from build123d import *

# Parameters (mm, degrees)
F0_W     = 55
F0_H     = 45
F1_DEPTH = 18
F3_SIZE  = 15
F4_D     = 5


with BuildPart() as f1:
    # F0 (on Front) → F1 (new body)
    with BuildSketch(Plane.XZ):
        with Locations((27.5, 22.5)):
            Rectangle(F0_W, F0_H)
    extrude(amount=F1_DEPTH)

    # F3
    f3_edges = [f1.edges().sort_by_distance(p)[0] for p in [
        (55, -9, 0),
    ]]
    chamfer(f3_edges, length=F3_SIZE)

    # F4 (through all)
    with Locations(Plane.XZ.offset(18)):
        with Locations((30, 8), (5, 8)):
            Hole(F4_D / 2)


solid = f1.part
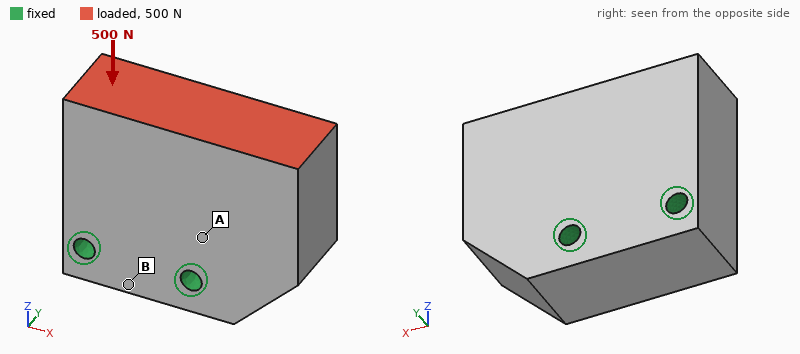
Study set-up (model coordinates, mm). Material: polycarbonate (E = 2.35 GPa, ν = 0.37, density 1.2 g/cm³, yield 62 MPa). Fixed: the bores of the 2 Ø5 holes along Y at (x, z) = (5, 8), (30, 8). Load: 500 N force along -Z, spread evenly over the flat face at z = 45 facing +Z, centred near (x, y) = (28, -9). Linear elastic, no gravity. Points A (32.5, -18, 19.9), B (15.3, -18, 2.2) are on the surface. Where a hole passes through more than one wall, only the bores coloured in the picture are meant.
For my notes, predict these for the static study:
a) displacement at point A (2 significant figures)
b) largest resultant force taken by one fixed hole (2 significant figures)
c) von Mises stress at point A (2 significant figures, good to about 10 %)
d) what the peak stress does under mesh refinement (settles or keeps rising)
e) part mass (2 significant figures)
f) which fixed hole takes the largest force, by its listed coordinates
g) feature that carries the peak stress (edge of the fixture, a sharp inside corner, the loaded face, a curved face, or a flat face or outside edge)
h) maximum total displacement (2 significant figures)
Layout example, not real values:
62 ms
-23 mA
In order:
8.6 µm
420 N
1.0 MPa
keeps rising
50 g
(30, 8)
edge of the fixture
30 µm
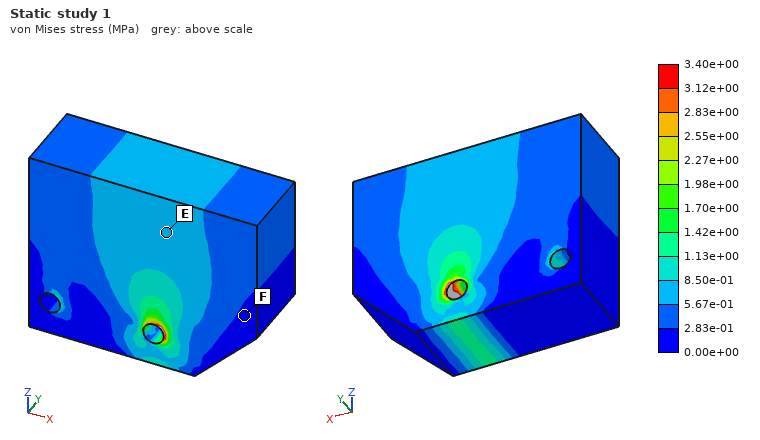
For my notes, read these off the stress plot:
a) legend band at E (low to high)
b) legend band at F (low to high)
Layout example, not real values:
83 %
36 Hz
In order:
5.67e-01 to 8.50e-01 MPa
0.00e+00 to 2.83e-01 MPa
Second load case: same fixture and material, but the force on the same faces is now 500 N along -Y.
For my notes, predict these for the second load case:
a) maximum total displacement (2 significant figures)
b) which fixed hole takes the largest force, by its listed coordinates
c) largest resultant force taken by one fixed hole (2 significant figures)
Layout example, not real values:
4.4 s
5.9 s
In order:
0.26 mm
(30, 8)
370 N
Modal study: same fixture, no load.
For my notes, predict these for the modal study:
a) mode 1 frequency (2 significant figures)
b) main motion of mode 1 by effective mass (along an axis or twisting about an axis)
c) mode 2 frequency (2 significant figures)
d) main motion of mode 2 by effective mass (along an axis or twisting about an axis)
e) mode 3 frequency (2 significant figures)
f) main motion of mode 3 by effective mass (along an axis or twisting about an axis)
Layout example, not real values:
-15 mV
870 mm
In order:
2000 Hz
along Y
2900 Hz
along X
3200 Hz
twisting about Z
